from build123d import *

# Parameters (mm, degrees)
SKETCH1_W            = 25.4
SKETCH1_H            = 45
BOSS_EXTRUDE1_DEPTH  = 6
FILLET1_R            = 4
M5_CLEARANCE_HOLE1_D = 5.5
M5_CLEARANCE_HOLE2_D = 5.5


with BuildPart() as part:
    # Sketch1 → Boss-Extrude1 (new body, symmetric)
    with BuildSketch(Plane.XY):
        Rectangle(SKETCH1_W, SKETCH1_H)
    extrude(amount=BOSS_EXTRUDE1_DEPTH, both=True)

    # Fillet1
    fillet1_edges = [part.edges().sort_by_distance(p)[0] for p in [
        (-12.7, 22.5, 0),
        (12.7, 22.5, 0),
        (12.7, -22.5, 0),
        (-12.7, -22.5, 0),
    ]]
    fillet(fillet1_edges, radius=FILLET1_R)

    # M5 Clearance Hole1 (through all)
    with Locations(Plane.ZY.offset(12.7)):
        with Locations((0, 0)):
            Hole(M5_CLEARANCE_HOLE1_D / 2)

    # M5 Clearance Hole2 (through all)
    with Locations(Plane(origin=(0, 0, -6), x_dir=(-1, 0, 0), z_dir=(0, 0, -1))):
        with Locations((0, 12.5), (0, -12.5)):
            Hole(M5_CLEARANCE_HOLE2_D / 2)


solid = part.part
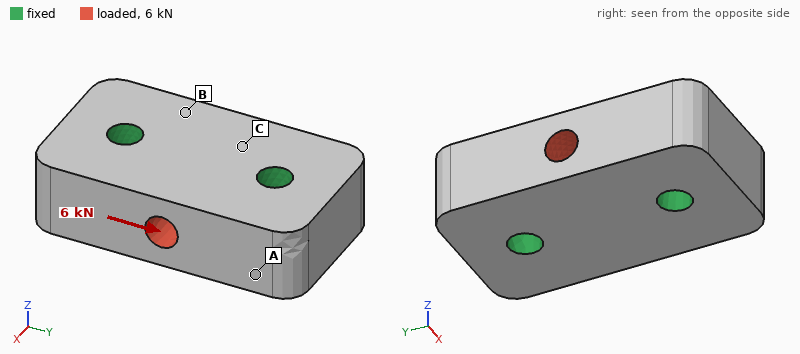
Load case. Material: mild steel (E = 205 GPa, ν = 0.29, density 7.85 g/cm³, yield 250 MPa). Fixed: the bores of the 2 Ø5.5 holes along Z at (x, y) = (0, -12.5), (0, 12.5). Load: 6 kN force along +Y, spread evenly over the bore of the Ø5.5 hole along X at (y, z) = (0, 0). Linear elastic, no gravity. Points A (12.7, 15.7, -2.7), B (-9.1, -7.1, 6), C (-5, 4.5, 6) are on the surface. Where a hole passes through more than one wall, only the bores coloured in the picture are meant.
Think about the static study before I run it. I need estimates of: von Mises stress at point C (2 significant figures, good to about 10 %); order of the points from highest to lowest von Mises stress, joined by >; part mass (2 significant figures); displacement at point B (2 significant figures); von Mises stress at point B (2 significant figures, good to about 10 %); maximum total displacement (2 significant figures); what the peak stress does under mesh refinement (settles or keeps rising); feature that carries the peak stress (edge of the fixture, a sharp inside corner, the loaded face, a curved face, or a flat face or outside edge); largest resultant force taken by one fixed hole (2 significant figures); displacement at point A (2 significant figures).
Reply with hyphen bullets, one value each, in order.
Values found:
- 9.1 MPa
- C > B > A
- 97 g
- 0.65 µm
- 5.6 MPa
- 0.98 µm
- keeps rising
- edge of the fixture
- 3.0 kN
- 0.56 µm
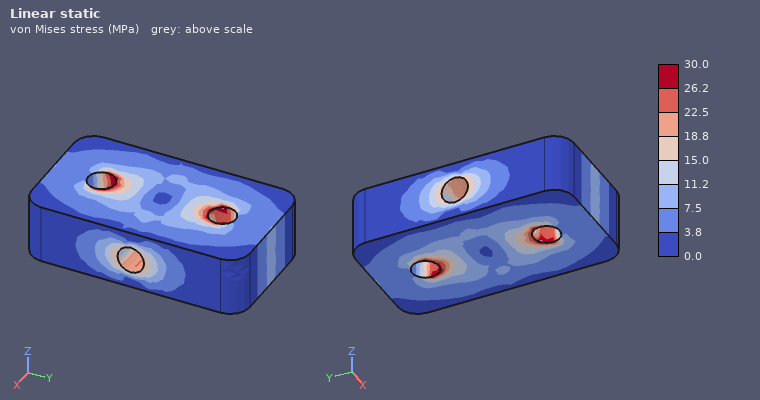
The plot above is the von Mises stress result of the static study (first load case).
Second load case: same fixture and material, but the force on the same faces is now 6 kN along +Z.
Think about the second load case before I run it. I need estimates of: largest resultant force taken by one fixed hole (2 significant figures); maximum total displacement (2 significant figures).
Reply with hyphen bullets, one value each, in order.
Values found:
- 3.0 kN
- 3.3 µm
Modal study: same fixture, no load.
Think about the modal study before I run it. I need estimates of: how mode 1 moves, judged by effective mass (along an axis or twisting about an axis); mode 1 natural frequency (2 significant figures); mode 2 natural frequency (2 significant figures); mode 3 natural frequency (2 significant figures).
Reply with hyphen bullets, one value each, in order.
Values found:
- twisting about Y
- 36 kHz
- 42 kHz
- 43 kHz
